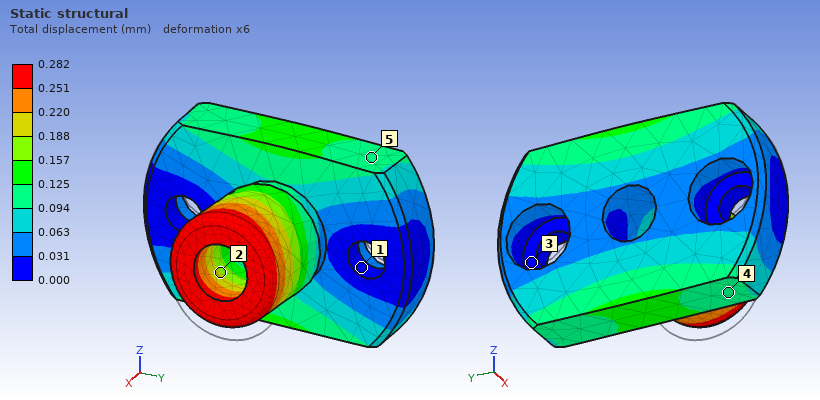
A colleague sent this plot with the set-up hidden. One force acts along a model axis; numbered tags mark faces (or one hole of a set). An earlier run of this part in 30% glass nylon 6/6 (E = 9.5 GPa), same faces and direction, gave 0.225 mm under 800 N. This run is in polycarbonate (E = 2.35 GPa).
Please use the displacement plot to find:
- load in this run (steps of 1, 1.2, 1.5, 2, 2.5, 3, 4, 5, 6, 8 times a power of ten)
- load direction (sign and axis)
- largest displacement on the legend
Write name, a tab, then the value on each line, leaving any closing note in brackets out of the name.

load in this run	250 N
load direction	+Z
largest displacement on the legend	0.282 mm
